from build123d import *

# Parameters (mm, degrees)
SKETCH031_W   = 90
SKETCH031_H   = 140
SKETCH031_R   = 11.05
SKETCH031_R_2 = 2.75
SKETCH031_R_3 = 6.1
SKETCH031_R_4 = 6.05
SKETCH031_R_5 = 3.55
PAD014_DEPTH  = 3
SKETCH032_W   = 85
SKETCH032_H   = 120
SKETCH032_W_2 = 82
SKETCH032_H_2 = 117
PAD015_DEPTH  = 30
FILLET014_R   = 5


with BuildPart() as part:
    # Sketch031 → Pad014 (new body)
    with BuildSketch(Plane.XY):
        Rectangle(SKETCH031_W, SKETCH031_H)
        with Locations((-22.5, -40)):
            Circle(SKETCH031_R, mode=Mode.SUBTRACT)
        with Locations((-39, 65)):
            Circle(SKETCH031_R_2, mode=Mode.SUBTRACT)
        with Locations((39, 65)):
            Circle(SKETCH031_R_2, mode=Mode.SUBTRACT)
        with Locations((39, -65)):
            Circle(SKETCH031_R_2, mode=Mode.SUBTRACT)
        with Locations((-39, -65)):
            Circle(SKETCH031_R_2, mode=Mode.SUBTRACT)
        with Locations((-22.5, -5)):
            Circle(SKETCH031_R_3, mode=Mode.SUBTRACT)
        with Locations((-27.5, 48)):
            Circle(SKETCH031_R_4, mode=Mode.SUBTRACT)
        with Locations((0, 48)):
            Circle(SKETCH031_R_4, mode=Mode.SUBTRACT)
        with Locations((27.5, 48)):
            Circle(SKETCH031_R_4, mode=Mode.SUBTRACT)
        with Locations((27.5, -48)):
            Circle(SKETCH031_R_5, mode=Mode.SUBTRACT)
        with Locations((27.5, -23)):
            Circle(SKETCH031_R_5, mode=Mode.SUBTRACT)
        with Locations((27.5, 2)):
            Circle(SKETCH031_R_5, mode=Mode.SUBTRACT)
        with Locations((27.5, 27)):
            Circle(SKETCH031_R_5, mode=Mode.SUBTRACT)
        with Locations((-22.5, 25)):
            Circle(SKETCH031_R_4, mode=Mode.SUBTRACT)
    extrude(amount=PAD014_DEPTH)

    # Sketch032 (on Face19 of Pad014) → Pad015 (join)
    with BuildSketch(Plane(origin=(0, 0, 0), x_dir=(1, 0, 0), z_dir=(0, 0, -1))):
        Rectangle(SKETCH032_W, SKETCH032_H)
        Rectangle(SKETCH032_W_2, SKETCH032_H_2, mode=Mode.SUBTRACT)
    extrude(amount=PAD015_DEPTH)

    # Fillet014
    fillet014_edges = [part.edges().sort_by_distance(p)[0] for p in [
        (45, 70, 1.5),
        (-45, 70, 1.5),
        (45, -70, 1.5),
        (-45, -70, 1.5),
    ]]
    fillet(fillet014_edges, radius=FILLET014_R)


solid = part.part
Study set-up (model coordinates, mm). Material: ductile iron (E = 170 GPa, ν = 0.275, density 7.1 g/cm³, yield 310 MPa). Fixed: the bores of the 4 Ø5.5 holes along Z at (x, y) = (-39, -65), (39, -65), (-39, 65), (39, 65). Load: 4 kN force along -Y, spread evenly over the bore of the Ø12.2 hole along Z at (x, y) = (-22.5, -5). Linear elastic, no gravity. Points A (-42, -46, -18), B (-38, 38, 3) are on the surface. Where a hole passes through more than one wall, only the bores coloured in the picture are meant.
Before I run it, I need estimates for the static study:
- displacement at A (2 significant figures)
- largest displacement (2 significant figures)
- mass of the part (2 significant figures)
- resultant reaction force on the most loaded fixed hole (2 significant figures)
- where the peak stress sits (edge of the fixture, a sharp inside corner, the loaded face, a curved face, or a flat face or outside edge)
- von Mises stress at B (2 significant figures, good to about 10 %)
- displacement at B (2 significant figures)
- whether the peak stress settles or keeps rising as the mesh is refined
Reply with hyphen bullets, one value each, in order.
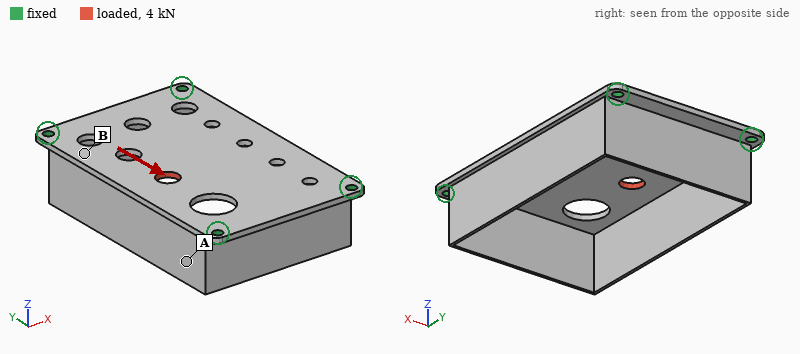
- 4.6 µm
- 9.7 µm
- 370 g
- 1.3 kN
- edge of the fixture
- 22 MPa
- 4.2 µm
- keeps rising
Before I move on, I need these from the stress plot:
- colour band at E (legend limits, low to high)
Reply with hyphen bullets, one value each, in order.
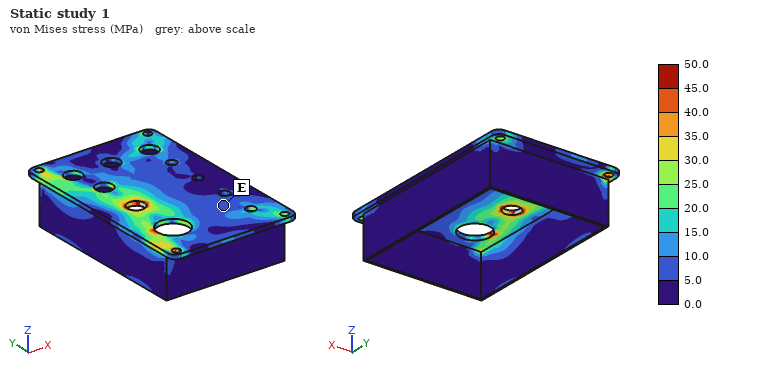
- 5.0 to 10.0 MPa
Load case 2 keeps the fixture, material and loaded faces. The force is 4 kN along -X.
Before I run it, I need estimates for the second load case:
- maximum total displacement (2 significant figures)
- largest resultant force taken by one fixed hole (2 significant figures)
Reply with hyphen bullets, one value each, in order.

- 18 µm
- 1.4 kN
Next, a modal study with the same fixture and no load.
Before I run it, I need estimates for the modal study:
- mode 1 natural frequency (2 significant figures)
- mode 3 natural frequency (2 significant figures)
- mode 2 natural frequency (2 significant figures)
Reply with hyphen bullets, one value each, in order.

- 1300 Hz
- 1700 Hz
- 1500 Hz
